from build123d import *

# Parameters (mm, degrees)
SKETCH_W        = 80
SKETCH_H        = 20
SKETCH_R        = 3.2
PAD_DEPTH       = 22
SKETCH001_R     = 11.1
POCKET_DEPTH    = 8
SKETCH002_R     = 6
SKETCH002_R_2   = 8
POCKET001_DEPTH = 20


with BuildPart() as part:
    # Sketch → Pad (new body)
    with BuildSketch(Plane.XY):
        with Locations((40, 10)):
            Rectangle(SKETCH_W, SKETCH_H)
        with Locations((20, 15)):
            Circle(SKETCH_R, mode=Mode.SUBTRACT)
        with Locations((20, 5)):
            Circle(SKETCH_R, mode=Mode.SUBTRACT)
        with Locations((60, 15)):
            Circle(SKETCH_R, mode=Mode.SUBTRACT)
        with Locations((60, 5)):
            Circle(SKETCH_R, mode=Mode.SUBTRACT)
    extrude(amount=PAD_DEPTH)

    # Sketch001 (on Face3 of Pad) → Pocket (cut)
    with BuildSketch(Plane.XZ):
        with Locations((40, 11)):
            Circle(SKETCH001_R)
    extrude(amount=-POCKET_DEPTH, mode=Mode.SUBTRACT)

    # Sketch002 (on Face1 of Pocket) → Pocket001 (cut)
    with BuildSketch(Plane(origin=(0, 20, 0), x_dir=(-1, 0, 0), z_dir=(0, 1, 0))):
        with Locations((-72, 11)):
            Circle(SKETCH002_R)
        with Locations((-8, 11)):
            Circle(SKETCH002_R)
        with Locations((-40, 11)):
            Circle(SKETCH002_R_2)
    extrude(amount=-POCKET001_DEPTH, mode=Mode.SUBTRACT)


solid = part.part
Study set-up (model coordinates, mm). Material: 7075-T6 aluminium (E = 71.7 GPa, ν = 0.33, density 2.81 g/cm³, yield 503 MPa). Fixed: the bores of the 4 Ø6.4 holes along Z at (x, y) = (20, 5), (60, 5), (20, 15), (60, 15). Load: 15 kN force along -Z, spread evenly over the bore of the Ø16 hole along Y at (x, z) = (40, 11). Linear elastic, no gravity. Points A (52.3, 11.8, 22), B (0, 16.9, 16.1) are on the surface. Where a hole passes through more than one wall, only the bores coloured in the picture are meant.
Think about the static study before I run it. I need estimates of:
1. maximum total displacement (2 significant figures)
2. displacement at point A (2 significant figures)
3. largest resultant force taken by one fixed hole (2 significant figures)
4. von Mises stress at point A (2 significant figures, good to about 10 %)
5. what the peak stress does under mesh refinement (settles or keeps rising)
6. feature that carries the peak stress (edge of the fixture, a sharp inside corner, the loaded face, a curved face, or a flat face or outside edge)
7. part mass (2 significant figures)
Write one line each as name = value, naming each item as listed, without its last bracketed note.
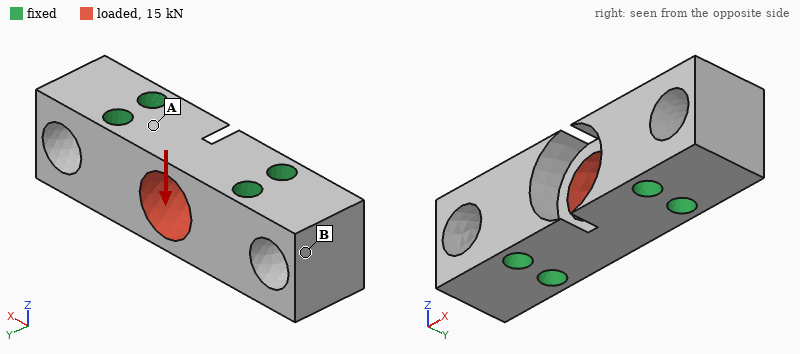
maximum total displacement = 32 µm
displacement at point A = 7.1 µm
largest resultant force taken by one fixed hole = 5.2 kN
von Mises stress at point A = 41 MPa
what the peak stress does under mesh refinement = keeps rising
feature that carries the peak stress = edge of the fixture
part mass = 63 g
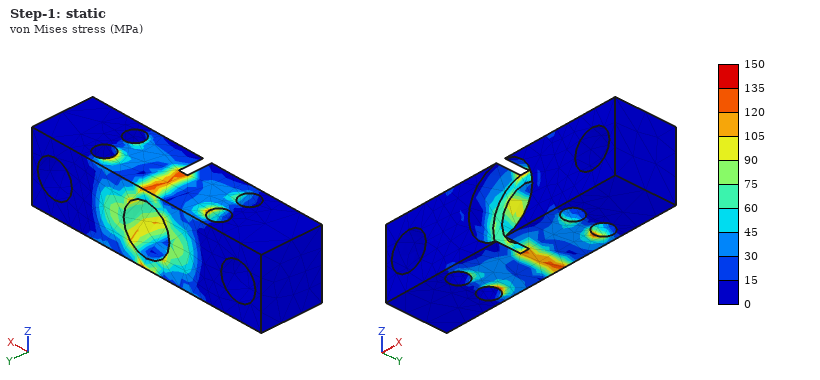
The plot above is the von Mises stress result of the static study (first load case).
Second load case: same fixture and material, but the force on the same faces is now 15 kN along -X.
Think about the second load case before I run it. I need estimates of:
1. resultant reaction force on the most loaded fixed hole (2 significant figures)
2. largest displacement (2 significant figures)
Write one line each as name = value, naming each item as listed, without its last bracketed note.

resultant reaction force on the most loaded fixed hole = 5.6 kN
largest displacement = 6.9 µm
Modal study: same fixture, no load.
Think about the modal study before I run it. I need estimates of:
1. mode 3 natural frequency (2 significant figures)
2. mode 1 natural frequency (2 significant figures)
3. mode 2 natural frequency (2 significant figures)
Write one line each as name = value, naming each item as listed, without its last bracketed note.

mode 3 natural frequency = 27 kHz
mode 1 natural frequency = 21 kHz
mode 2 natural frequency = 21 kHz
